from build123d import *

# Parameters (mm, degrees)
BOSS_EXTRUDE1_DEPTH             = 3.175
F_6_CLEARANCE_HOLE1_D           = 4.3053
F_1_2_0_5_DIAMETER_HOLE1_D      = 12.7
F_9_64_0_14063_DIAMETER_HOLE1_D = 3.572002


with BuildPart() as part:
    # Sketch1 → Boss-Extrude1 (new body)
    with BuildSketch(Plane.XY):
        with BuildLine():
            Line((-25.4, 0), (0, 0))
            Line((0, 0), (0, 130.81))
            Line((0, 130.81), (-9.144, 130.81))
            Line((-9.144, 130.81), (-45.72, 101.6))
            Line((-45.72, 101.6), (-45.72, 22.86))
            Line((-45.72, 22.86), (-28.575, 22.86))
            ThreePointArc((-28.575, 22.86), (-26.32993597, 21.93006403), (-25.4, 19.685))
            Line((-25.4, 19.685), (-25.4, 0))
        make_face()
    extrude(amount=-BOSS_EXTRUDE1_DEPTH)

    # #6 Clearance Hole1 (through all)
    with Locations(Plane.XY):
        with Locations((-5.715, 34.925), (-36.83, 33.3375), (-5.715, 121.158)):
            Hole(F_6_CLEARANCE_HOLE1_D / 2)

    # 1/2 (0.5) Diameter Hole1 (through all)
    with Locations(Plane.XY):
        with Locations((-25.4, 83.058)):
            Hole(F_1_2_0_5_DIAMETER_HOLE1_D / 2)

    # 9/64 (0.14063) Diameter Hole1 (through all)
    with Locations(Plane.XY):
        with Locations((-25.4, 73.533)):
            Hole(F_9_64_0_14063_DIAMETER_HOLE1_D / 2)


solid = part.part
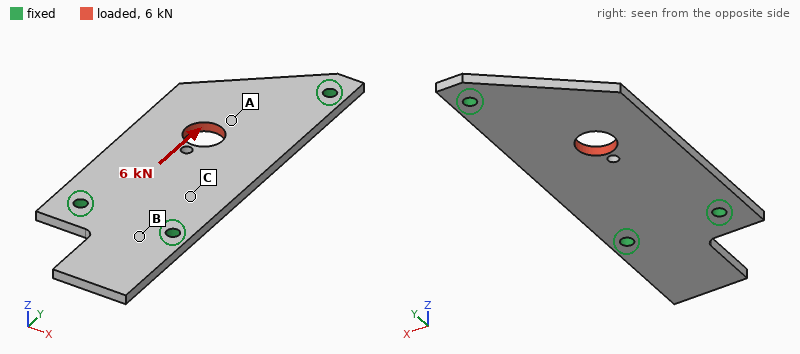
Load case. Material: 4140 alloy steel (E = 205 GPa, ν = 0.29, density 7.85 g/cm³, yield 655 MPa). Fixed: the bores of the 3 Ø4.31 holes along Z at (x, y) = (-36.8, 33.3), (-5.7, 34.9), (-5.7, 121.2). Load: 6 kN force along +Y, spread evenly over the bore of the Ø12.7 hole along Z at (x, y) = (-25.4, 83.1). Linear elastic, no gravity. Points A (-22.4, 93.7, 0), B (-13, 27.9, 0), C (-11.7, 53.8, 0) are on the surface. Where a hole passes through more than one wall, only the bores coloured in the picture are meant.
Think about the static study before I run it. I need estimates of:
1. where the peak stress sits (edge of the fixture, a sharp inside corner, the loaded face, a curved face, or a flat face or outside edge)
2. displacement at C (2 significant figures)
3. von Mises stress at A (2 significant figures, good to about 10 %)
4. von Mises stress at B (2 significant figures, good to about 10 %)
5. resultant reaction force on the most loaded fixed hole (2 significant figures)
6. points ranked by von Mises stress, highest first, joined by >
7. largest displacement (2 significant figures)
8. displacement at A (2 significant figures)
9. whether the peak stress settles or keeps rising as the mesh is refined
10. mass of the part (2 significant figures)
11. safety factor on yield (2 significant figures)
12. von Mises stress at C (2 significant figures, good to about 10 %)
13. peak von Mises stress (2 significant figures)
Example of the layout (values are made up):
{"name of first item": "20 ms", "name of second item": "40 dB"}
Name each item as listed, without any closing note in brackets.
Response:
{"where the peak stress sits": "a curved face", "displacement at C": "3.5 µm", "von Mises stress at A": "44 MPa", "von Mises stress at B": "12 MPa", "resultant reaction force on the most loaded fixed hole": "2.2 kN", "points ranked by von Mises stress, highest first, joined by >": "A > C > B", "largest displacement": "11 µm", "displacement at A": "8.7 µm", "whether the peak stress settles or keeps rising as the mesh is refined": "settles", "mass of the part": "120 g", "safety factor on yield": "3.6", "von Mises stress at C": "29 MPa", "peak von Mises stress": "180 MPa"}
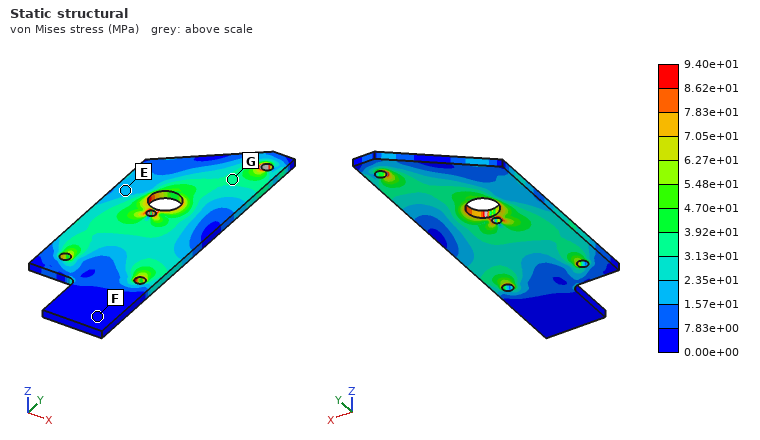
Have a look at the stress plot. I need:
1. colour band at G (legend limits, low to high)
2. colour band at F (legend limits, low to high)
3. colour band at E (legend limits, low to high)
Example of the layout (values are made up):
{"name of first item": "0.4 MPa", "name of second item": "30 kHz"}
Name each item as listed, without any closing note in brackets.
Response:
{"colour band at G": "3.13e+01 to 3.92e+01 MPa", "colour band at F": "0.00e+00 to 7.83e+00 MPa", "colour band at E": "1.57e+01 to 2.35e+01 MPa"}
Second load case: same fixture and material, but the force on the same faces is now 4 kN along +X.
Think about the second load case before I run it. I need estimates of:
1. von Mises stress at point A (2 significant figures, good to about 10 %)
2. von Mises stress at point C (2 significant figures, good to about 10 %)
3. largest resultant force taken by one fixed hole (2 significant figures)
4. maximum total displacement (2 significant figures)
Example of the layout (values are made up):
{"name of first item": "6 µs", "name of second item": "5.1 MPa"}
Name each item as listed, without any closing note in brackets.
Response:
{"von Mises stress at point A": "25 MPa", "von Mises stress at point C": "32 MPa", "largest resultant force taken by one fixed hole": "2.2 kN", "maximum total displacement": "15 µm"}
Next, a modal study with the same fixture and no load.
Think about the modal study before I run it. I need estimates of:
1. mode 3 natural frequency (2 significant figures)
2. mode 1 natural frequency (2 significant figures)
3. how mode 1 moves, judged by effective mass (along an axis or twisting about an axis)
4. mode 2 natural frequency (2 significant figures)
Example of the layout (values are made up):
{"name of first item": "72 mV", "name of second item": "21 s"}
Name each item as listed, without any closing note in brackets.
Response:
{"mode 3 natural frequency": "2800 Hz", "mode 1 natural frequency": "1600 Hz", "how mode 1 moves, judged by effective mass": "along Z", "mode 2 natural frequency": "2300 Hz"}
